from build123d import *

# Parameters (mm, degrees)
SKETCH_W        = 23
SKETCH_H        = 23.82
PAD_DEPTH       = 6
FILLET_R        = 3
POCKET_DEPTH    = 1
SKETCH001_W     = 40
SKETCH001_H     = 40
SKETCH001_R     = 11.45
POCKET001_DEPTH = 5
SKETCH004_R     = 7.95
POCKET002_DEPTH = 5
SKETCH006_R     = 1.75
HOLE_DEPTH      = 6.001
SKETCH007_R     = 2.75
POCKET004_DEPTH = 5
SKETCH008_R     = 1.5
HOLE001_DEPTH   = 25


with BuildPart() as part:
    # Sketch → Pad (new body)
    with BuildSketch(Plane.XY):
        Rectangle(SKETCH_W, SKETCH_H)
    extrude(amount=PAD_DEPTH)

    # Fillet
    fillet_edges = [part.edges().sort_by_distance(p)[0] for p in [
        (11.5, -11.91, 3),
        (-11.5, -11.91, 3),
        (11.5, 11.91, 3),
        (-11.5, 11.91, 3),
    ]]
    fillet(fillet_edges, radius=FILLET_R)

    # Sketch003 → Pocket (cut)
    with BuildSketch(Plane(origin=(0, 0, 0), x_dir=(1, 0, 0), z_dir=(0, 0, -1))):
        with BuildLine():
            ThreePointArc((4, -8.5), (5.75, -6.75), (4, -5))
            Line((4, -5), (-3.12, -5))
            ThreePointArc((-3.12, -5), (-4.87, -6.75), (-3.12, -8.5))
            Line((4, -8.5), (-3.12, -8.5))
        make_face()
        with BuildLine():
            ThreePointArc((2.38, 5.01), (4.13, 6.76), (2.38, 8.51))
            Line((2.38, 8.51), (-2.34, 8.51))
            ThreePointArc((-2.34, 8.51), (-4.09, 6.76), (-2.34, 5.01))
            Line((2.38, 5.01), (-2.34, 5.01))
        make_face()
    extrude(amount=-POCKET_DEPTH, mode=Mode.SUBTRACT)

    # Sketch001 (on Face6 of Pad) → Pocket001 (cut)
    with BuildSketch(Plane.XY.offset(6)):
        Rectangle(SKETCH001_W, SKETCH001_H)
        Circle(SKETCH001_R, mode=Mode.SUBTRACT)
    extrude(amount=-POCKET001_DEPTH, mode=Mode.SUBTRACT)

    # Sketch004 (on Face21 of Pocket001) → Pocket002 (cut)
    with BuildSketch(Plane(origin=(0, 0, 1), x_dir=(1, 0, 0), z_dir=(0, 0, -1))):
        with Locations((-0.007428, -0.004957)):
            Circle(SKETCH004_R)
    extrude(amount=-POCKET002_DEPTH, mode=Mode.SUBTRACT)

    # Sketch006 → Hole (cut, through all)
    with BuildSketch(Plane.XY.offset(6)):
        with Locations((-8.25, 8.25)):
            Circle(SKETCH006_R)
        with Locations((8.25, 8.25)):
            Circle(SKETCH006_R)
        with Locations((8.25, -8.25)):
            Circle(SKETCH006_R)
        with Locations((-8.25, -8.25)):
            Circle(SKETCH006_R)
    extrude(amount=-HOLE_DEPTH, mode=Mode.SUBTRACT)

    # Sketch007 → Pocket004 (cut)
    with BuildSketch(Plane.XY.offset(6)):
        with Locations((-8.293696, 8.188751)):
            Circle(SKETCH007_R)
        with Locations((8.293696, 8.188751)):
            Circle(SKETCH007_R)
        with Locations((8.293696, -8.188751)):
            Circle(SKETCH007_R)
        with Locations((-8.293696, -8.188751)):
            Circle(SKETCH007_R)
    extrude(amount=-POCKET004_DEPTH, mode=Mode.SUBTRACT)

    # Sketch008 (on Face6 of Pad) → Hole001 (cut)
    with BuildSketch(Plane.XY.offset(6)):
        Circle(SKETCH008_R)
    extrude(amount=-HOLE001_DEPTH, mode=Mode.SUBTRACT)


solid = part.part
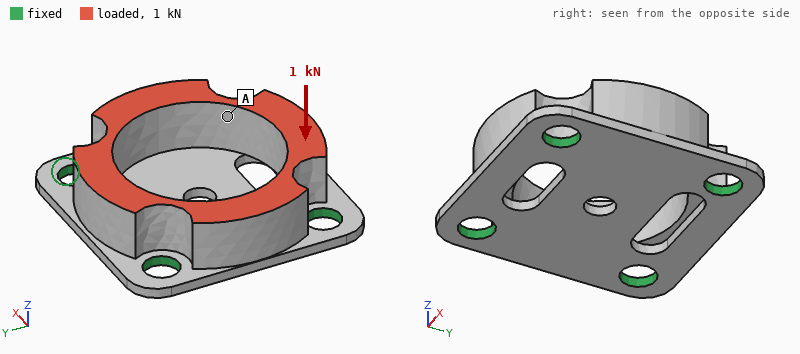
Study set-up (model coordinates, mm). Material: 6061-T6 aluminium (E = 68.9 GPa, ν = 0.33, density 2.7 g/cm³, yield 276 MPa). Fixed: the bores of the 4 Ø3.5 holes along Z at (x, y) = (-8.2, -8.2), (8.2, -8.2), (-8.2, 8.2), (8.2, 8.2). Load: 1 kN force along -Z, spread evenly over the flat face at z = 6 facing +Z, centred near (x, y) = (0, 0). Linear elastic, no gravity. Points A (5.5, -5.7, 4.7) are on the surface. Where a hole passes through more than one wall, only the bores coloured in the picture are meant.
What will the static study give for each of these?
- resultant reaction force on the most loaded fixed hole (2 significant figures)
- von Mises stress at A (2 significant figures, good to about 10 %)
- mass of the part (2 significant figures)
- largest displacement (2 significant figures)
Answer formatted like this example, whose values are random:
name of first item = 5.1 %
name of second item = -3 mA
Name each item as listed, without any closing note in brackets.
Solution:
resultant reaction force on the most loaded fixed hole = 260 N
von Mises stress at A = 16 MPa
mass of the part = 3.5 g
largest displacement = 5.5 µm
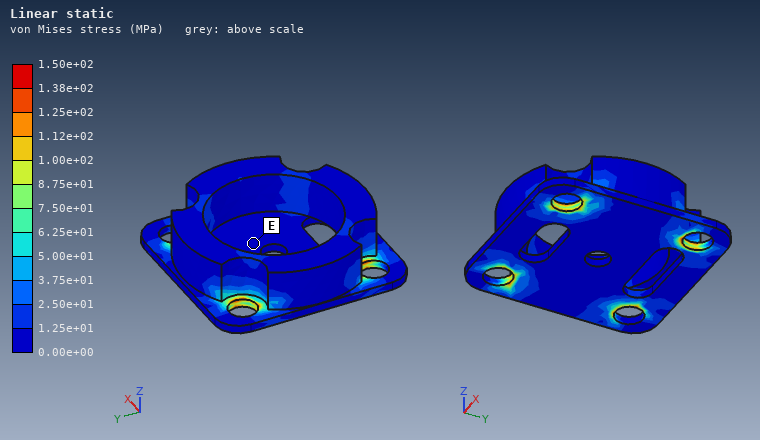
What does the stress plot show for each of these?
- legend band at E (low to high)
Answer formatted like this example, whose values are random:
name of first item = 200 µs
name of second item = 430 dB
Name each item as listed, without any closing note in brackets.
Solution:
legend band at E = 0.00e+00 to 1.25e+01 MPa
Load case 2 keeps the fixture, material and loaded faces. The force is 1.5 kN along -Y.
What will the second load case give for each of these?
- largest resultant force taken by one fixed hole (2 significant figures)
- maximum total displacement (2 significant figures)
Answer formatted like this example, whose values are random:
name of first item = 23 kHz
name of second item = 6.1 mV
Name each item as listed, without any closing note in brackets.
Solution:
largest resultant force taken by one fixed hole = 460 N
maximum total displacement = 22 µm
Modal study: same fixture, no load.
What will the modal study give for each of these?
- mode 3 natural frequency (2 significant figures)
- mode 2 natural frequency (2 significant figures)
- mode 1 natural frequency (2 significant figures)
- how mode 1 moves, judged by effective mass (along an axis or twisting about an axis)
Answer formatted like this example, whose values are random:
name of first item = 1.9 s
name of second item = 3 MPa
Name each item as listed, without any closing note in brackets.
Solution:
mode 3 natural frequency = 39 kHz
mode 2 natural frequency = 30 kHz
mode 1 natural frequency = 25 kHz
how mode 1 moves, judged by effective mass = along Z
